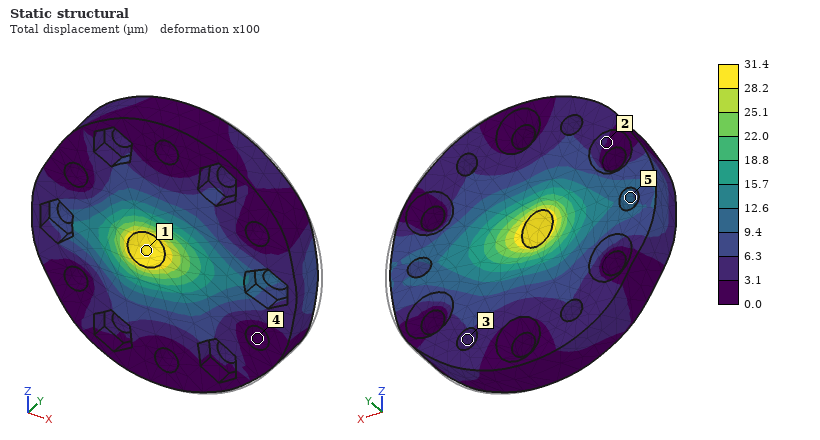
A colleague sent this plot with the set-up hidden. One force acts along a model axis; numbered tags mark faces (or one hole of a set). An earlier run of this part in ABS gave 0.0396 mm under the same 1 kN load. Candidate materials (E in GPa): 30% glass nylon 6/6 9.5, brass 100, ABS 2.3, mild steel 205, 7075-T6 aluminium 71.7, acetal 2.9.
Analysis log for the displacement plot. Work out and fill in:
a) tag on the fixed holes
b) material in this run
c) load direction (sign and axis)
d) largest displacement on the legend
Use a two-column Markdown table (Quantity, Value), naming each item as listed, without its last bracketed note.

| Quantity | Value |
|---|---|
| tag on the fixed holes | 4 |
| material in this run | acetal |
| load direction | -X |
| largest displacement on the legend | 31.4 µm |
